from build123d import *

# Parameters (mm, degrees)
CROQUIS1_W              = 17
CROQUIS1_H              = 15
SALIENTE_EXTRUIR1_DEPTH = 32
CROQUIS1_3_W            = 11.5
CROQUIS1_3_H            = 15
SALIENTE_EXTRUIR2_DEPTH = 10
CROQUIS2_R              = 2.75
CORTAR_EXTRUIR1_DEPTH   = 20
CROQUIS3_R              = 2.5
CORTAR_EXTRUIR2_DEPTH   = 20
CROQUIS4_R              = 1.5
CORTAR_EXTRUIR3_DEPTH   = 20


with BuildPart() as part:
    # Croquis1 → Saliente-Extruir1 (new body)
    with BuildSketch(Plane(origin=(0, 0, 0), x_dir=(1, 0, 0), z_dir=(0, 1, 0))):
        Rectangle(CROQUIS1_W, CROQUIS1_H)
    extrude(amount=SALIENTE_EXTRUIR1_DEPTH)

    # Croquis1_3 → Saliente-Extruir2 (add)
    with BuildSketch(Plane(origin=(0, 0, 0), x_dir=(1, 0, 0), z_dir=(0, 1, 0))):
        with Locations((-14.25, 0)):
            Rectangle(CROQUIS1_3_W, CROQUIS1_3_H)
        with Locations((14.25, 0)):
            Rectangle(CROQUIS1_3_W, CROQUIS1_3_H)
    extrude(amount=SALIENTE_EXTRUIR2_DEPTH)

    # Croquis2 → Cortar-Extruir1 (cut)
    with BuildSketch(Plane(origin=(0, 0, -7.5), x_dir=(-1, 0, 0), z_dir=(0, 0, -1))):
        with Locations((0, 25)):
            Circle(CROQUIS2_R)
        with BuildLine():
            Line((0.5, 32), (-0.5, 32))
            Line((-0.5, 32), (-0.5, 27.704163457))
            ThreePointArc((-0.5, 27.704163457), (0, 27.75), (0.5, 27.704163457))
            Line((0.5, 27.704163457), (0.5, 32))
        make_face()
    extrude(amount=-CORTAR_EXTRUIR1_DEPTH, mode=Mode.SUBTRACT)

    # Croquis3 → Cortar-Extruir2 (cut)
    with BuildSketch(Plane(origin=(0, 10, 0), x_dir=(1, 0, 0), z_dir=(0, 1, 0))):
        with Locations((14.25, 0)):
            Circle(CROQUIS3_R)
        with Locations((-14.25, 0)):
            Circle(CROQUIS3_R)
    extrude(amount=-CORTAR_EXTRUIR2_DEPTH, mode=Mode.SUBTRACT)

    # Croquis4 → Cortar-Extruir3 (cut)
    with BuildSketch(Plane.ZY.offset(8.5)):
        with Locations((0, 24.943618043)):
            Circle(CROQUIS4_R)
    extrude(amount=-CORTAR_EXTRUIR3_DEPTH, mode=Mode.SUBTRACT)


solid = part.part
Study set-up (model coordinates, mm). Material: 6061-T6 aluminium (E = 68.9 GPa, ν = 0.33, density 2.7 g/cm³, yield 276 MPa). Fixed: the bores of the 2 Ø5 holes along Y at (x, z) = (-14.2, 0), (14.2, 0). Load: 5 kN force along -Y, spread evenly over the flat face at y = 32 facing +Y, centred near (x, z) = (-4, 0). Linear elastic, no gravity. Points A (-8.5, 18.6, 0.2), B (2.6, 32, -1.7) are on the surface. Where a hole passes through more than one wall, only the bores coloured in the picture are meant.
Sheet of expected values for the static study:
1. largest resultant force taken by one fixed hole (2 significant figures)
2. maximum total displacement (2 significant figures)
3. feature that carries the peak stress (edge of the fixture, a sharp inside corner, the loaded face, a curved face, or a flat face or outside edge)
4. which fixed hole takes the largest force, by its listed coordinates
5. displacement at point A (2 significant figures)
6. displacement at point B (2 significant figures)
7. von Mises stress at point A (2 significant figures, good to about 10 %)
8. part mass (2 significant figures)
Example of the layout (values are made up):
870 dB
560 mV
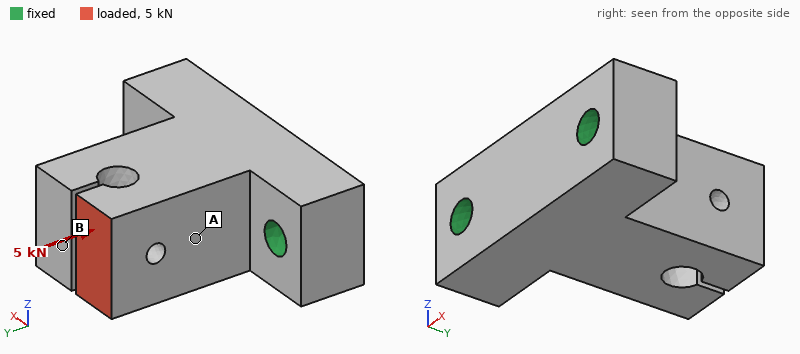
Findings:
3.5 kN
32 µm
a curved face
(-14.2, 0)
17 µm
17 µm
38 MPa
29 g
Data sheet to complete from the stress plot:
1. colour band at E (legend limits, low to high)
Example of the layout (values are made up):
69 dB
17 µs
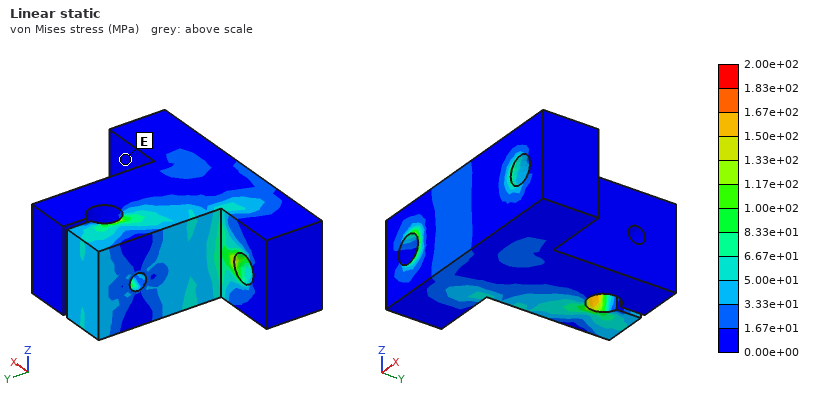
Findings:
0.00e+00 to 1.67e+01 MPa
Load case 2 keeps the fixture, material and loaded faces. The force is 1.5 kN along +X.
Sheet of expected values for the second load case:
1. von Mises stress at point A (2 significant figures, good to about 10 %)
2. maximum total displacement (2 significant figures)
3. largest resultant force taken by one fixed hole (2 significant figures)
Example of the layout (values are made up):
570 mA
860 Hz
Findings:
74 MPa
90 µm
1.9 kN
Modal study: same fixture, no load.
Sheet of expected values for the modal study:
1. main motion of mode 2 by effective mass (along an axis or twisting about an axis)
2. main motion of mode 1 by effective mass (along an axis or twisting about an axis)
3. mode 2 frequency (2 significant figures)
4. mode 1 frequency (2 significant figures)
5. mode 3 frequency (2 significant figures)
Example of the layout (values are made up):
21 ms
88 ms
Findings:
along X
along Z
15 kHz
9200 Hz
24 kHz
